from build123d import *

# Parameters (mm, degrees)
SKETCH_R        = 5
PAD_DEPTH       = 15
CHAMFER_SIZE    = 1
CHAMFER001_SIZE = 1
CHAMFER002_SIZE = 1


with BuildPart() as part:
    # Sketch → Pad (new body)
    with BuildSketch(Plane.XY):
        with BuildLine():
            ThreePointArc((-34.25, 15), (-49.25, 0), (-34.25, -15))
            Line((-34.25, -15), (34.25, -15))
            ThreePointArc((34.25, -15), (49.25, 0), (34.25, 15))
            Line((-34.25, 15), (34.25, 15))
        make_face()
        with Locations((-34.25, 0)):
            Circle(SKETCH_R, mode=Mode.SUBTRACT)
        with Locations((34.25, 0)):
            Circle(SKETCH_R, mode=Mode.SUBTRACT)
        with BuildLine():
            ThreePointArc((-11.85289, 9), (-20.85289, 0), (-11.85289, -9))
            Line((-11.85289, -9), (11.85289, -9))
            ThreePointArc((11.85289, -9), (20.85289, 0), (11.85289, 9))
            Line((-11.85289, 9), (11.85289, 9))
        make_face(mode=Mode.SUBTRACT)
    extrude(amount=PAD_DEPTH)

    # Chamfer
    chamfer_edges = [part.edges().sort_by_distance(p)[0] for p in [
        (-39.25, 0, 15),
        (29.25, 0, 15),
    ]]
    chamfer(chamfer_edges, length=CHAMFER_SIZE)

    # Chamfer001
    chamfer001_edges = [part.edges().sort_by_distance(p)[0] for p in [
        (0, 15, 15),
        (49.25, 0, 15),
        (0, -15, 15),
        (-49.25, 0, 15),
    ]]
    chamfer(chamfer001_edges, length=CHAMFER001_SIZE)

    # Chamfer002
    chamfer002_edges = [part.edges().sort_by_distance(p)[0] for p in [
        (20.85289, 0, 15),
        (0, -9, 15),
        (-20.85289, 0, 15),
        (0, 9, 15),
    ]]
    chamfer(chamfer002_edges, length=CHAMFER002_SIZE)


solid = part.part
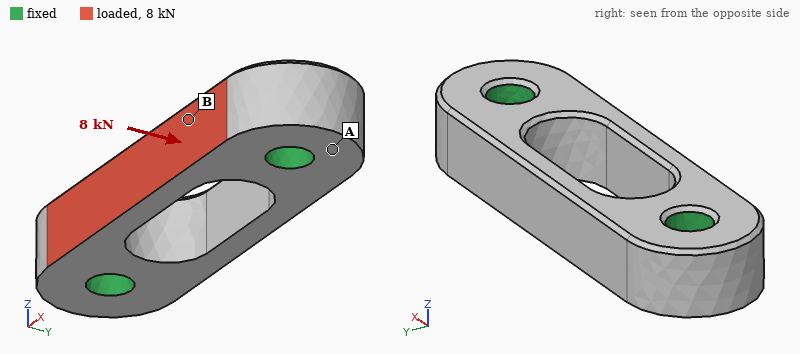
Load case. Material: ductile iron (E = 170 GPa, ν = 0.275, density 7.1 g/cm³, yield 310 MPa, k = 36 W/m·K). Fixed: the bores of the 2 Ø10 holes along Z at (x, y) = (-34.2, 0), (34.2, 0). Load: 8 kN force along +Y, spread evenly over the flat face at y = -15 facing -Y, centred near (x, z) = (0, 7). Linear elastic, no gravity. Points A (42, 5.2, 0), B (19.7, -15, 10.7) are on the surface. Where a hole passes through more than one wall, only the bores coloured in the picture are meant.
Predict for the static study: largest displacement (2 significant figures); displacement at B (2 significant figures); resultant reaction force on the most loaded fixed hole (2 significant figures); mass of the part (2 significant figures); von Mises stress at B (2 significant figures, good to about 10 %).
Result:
25 µm
6.1 µm
4.3 kN
200 g
43 MPa
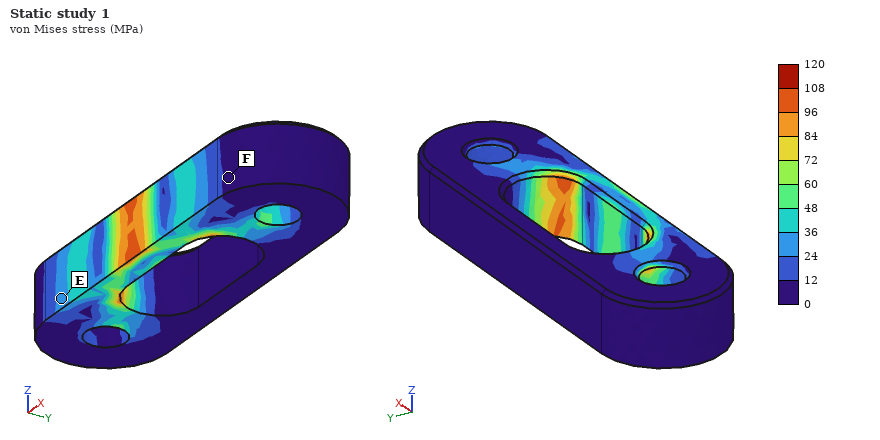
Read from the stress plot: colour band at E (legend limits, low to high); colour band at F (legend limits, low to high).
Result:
24 to 36 MPa
0 to 12 MPa
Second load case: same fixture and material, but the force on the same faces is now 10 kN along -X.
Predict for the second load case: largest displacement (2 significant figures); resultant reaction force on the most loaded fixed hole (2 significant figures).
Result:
7.5 µm
5.1 kN
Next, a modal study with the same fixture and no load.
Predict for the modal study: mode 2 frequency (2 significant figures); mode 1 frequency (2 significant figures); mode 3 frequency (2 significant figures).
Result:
16 kHz
15 kHz
16 kHz
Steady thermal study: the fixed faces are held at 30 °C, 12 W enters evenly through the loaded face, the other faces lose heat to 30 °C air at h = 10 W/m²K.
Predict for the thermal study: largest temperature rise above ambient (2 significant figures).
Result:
19 K
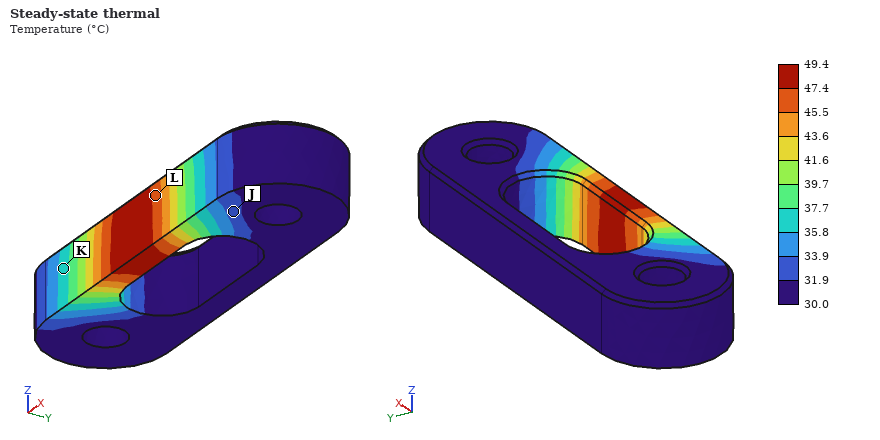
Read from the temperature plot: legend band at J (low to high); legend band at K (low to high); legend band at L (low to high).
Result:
31.9 to 33.9 °C
35.8 to 37.7 °C
45.5 to 47.4 °C
